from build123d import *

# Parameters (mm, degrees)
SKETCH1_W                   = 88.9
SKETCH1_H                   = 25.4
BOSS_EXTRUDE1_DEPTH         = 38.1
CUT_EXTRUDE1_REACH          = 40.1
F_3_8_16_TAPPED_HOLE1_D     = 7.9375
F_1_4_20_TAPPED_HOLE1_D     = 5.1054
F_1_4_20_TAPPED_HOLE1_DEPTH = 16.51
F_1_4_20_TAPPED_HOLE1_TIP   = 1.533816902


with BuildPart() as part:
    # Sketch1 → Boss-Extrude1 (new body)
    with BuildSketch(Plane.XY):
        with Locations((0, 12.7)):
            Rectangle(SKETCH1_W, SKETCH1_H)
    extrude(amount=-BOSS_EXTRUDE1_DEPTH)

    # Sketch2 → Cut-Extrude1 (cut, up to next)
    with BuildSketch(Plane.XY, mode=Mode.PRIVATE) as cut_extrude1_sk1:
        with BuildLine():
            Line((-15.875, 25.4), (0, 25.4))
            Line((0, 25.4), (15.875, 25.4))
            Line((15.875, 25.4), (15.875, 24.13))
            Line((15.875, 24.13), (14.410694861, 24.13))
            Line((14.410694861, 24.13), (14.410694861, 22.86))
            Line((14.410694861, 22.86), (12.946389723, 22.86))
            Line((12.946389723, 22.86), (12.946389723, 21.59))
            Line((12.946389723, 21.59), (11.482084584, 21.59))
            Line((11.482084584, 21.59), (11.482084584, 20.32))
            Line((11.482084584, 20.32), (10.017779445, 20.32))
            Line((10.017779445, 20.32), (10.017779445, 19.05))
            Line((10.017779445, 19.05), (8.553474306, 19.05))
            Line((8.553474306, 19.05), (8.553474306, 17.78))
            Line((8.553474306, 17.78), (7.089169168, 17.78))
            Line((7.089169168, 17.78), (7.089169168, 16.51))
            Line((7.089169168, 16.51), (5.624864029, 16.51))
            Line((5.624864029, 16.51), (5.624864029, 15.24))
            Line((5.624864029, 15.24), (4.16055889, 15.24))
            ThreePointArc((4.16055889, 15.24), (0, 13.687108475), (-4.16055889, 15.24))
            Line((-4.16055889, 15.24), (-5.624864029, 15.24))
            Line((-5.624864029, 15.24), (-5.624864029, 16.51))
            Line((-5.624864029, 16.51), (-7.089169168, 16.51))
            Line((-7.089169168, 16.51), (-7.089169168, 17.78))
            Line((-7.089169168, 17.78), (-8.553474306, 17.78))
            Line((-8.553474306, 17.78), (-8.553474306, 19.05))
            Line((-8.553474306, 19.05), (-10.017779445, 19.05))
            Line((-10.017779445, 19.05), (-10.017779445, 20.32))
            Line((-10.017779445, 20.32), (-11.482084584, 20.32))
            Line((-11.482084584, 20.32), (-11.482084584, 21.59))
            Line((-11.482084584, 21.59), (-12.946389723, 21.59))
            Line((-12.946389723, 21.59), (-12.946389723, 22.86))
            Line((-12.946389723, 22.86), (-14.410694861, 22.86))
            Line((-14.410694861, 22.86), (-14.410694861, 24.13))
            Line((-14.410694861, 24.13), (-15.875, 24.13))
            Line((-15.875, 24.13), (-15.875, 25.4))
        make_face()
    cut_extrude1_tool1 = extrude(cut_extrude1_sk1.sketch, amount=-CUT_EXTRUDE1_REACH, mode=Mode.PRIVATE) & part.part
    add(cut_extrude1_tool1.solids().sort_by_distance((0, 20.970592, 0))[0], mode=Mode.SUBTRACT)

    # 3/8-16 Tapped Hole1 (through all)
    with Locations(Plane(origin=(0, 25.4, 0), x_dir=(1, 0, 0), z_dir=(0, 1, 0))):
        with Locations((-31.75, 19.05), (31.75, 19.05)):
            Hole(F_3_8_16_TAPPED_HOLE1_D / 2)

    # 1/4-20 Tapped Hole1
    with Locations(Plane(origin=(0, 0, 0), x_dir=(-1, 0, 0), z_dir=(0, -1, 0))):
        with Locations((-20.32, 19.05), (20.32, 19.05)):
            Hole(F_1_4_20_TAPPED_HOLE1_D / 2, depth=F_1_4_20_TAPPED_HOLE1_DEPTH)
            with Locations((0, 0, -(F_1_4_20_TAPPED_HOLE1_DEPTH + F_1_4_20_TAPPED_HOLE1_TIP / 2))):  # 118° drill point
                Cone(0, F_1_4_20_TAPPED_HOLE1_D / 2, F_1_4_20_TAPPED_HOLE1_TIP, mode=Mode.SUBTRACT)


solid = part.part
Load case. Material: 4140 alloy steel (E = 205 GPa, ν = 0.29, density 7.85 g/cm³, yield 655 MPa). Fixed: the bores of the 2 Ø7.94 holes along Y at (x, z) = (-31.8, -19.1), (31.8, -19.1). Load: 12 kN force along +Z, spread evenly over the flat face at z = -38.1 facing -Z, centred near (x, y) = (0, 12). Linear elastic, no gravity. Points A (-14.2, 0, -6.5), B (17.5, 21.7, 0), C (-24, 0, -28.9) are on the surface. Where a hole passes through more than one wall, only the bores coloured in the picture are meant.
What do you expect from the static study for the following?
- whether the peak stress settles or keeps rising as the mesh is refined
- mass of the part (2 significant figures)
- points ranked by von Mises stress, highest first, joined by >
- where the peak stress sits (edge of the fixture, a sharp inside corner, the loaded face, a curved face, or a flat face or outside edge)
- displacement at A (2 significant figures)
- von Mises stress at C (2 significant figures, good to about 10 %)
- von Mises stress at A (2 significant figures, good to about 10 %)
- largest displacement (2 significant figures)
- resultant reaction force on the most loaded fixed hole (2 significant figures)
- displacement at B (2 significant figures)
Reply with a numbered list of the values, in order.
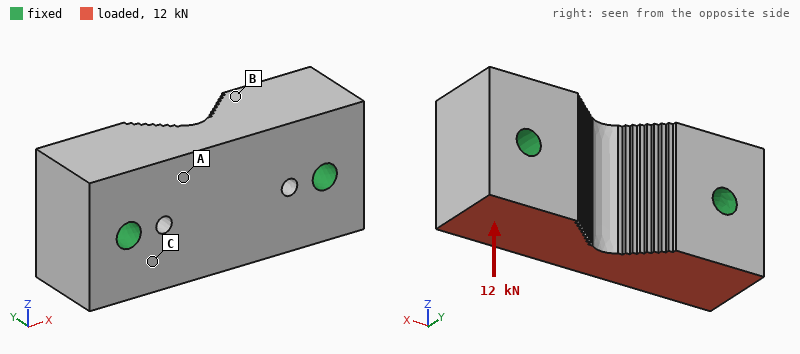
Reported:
1. keeps rising
2. 580 g
3. C > A > B
4. edge of the fixture
5. 1.4 µm
6. 11 MPa
7. 6.6 MPa
8. 2.5 µm
9. 6.0 kN
10. 1.1 µm
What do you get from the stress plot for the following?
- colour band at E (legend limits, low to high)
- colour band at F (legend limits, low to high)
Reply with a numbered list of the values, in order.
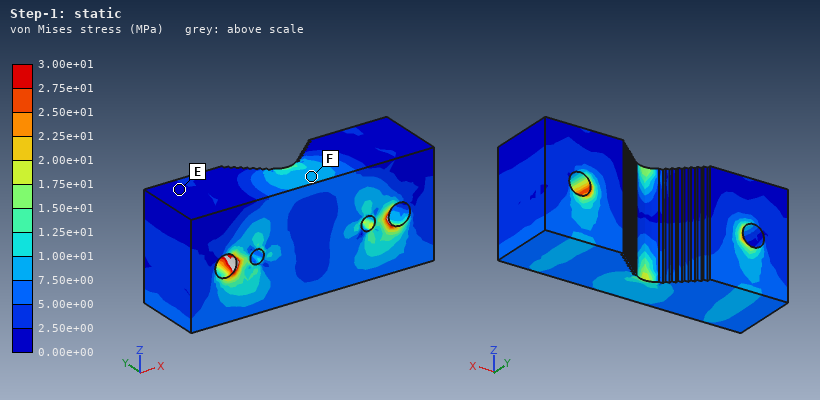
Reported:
1. 0.00e+00 to 2.50e+00 MPa
2. 7.50e+00 to 1.00e+01 MPa
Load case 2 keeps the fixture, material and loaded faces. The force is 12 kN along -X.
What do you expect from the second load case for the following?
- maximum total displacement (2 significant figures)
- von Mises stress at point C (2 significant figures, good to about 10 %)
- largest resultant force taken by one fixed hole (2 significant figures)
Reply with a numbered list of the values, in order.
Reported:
1. 3.6 µm
2. 15 MPa
3. 6.6 kN
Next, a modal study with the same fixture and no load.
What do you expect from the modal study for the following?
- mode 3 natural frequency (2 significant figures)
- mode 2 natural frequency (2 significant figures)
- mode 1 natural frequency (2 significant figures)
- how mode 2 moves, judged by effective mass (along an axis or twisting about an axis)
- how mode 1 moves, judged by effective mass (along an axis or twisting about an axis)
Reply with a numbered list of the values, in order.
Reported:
1. 22 kHz
2. 17 kHz
3. 16 kHz
4. along Y
5. along Z
